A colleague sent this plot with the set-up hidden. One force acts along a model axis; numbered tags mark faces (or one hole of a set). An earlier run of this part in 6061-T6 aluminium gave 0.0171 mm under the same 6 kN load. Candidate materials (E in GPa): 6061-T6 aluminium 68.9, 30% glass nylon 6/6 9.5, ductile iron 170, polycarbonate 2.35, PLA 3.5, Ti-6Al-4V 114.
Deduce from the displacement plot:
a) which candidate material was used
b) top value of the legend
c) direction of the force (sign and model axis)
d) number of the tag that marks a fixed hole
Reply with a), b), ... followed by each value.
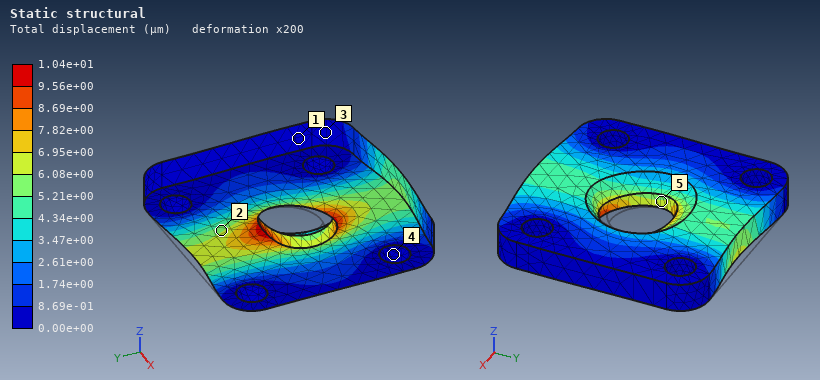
a) Ti-6Al-4V
b) 1.04e+01 µm
c) -Y
d) 4
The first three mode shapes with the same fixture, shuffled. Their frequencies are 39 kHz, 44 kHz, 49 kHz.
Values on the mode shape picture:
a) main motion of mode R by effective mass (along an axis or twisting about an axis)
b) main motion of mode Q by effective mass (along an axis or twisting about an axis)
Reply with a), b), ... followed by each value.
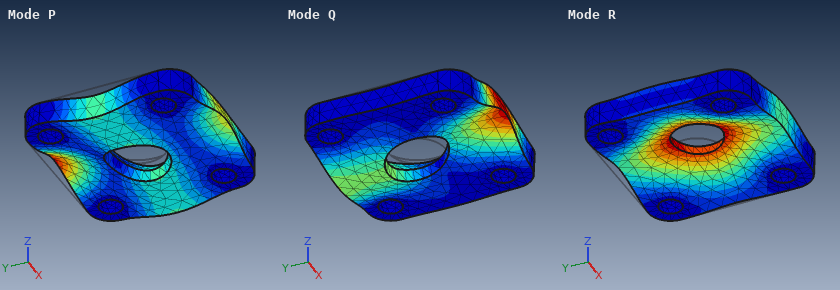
a) along Z
b) twisting about X
